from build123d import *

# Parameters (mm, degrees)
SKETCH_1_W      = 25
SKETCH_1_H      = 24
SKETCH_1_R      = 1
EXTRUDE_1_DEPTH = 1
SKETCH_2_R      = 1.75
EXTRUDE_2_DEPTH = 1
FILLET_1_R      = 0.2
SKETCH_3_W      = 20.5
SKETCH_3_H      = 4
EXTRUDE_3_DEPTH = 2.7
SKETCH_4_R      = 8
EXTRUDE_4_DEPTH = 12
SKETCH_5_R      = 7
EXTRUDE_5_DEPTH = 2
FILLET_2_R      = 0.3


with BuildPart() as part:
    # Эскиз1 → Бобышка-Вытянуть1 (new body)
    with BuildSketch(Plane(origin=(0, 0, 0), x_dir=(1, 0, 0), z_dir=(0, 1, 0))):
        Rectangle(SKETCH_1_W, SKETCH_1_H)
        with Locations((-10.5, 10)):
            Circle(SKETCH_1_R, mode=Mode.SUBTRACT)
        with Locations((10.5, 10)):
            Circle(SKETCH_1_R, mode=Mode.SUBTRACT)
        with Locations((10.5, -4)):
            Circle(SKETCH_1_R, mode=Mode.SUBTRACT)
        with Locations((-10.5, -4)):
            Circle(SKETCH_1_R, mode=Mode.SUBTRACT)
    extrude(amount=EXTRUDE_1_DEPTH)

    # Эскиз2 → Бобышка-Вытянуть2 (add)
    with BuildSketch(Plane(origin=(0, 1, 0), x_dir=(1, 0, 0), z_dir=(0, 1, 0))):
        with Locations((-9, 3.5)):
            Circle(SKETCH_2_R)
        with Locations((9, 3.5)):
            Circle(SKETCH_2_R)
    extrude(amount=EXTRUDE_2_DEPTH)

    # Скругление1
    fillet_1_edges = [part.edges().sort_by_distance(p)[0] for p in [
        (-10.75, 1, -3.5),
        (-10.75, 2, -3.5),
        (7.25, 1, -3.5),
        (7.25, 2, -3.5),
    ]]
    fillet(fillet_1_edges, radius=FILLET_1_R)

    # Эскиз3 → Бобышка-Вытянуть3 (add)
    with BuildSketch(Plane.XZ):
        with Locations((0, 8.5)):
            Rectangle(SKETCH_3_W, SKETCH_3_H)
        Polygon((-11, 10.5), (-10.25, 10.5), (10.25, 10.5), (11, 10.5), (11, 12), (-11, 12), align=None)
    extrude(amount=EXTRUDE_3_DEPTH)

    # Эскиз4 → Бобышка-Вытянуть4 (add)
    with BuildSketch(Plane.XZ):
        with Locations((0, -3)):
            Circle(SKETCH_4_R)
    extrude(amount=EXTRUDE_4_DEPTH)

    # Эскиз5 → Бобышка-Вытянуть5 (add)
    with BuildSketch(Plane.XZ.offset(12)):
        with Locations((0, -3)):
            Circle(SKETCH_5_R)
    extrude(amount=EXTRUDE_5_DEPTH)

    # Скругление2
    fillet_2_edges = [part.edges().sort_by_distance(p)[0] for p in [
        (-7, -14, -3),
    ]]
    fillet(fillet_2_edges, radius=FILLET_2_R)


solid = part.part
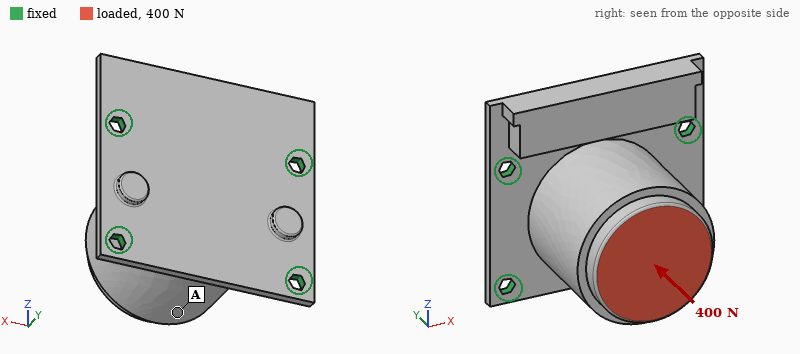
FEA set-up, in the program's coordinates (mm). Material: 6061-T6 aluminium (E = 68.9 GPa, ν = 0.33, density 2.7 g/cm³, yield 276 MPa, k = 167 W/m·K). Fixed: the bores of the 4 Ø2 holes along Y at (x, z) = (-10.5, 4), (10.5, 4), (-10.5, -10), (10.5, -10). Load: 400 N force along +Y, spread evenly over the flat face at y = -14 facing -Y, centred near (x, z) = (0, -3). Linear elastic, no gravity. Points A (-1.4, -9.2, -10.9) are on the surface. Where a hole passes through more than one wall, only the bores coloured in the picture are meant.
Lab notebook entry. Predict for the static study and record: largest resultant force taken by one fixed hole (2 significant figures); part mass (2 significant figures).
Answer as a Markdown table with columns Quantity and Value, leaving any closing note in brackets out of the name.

| Quantity | Value |
|---|---|
| largest resultant force taken by one fixed hole | 110 N |
| part mass | 9.8 g |
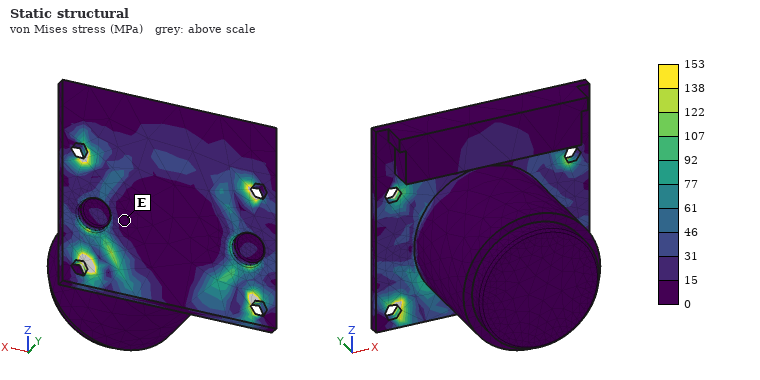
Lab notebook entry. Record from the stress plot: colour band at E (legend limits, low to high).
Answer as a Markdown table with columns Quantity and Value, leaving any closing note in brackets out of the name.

| Quantity | Value |
|---|---|
| colour band at E | 0 to 15 MPa |
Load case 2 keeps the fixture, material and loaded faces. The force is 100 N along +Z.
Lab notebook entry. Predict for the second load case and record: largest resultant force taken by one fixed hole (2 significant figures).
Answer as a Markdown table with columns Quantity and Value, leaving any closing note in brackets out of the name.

| Quantity | Value |
|---|---|
| largest resultant force taken by one fixed hole | 70 N |
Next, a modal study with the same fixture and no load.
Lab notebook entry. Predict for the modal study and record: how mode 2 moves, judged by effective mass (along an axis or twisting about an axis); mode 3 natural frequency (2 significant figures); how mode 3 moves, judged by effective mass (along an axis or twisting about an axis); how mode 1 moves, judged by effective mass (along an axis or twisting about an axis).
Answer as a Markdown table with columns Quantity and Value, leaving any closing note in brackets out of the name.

| Quantity | Value |
|---|---|
| how mode 2 moves, judged by effective mass | along X |
| mode 3 natural frequency | 8000 Hz |
| how mode 3 moves, judged by effective mass | along Y |
| how mode 1 moves, judged by effective mass | along Z |
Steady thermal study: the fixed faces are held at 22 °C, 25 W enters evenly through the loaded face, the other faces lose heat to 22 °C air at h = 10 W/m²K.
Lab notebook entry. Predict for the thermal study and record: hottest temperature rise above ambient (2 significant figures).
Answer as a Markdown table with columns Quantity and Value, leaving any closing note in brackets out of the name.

| Quantity | Value |
|---|---|
| hottest temperature rise above ambient | 34 K |
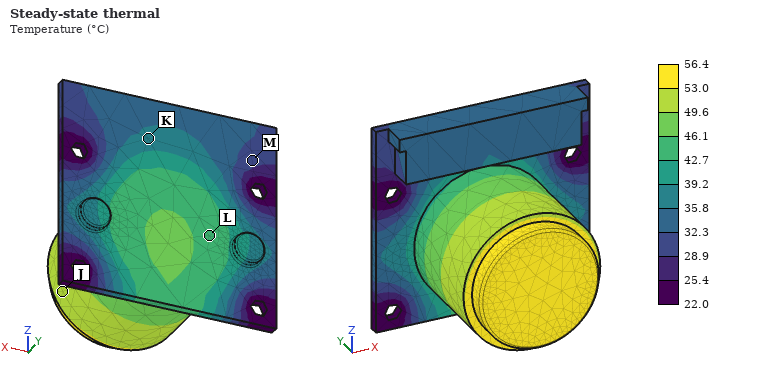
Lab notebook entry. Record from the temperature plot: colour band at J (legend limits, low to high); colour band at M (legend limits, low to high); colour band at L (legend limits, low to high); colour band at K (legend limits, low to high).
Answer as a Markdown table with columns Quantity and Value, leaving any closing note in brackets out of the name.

| Quantity | Value |
|---|---|
| colour band at J | 49.6 to 53.0 °C |
| colour band at M | 28.9 to 32.3 °C |
| colour band at L | 42.7 to 46.1 °C |
| colour band at K | 35.8 to 39.2 °C |
